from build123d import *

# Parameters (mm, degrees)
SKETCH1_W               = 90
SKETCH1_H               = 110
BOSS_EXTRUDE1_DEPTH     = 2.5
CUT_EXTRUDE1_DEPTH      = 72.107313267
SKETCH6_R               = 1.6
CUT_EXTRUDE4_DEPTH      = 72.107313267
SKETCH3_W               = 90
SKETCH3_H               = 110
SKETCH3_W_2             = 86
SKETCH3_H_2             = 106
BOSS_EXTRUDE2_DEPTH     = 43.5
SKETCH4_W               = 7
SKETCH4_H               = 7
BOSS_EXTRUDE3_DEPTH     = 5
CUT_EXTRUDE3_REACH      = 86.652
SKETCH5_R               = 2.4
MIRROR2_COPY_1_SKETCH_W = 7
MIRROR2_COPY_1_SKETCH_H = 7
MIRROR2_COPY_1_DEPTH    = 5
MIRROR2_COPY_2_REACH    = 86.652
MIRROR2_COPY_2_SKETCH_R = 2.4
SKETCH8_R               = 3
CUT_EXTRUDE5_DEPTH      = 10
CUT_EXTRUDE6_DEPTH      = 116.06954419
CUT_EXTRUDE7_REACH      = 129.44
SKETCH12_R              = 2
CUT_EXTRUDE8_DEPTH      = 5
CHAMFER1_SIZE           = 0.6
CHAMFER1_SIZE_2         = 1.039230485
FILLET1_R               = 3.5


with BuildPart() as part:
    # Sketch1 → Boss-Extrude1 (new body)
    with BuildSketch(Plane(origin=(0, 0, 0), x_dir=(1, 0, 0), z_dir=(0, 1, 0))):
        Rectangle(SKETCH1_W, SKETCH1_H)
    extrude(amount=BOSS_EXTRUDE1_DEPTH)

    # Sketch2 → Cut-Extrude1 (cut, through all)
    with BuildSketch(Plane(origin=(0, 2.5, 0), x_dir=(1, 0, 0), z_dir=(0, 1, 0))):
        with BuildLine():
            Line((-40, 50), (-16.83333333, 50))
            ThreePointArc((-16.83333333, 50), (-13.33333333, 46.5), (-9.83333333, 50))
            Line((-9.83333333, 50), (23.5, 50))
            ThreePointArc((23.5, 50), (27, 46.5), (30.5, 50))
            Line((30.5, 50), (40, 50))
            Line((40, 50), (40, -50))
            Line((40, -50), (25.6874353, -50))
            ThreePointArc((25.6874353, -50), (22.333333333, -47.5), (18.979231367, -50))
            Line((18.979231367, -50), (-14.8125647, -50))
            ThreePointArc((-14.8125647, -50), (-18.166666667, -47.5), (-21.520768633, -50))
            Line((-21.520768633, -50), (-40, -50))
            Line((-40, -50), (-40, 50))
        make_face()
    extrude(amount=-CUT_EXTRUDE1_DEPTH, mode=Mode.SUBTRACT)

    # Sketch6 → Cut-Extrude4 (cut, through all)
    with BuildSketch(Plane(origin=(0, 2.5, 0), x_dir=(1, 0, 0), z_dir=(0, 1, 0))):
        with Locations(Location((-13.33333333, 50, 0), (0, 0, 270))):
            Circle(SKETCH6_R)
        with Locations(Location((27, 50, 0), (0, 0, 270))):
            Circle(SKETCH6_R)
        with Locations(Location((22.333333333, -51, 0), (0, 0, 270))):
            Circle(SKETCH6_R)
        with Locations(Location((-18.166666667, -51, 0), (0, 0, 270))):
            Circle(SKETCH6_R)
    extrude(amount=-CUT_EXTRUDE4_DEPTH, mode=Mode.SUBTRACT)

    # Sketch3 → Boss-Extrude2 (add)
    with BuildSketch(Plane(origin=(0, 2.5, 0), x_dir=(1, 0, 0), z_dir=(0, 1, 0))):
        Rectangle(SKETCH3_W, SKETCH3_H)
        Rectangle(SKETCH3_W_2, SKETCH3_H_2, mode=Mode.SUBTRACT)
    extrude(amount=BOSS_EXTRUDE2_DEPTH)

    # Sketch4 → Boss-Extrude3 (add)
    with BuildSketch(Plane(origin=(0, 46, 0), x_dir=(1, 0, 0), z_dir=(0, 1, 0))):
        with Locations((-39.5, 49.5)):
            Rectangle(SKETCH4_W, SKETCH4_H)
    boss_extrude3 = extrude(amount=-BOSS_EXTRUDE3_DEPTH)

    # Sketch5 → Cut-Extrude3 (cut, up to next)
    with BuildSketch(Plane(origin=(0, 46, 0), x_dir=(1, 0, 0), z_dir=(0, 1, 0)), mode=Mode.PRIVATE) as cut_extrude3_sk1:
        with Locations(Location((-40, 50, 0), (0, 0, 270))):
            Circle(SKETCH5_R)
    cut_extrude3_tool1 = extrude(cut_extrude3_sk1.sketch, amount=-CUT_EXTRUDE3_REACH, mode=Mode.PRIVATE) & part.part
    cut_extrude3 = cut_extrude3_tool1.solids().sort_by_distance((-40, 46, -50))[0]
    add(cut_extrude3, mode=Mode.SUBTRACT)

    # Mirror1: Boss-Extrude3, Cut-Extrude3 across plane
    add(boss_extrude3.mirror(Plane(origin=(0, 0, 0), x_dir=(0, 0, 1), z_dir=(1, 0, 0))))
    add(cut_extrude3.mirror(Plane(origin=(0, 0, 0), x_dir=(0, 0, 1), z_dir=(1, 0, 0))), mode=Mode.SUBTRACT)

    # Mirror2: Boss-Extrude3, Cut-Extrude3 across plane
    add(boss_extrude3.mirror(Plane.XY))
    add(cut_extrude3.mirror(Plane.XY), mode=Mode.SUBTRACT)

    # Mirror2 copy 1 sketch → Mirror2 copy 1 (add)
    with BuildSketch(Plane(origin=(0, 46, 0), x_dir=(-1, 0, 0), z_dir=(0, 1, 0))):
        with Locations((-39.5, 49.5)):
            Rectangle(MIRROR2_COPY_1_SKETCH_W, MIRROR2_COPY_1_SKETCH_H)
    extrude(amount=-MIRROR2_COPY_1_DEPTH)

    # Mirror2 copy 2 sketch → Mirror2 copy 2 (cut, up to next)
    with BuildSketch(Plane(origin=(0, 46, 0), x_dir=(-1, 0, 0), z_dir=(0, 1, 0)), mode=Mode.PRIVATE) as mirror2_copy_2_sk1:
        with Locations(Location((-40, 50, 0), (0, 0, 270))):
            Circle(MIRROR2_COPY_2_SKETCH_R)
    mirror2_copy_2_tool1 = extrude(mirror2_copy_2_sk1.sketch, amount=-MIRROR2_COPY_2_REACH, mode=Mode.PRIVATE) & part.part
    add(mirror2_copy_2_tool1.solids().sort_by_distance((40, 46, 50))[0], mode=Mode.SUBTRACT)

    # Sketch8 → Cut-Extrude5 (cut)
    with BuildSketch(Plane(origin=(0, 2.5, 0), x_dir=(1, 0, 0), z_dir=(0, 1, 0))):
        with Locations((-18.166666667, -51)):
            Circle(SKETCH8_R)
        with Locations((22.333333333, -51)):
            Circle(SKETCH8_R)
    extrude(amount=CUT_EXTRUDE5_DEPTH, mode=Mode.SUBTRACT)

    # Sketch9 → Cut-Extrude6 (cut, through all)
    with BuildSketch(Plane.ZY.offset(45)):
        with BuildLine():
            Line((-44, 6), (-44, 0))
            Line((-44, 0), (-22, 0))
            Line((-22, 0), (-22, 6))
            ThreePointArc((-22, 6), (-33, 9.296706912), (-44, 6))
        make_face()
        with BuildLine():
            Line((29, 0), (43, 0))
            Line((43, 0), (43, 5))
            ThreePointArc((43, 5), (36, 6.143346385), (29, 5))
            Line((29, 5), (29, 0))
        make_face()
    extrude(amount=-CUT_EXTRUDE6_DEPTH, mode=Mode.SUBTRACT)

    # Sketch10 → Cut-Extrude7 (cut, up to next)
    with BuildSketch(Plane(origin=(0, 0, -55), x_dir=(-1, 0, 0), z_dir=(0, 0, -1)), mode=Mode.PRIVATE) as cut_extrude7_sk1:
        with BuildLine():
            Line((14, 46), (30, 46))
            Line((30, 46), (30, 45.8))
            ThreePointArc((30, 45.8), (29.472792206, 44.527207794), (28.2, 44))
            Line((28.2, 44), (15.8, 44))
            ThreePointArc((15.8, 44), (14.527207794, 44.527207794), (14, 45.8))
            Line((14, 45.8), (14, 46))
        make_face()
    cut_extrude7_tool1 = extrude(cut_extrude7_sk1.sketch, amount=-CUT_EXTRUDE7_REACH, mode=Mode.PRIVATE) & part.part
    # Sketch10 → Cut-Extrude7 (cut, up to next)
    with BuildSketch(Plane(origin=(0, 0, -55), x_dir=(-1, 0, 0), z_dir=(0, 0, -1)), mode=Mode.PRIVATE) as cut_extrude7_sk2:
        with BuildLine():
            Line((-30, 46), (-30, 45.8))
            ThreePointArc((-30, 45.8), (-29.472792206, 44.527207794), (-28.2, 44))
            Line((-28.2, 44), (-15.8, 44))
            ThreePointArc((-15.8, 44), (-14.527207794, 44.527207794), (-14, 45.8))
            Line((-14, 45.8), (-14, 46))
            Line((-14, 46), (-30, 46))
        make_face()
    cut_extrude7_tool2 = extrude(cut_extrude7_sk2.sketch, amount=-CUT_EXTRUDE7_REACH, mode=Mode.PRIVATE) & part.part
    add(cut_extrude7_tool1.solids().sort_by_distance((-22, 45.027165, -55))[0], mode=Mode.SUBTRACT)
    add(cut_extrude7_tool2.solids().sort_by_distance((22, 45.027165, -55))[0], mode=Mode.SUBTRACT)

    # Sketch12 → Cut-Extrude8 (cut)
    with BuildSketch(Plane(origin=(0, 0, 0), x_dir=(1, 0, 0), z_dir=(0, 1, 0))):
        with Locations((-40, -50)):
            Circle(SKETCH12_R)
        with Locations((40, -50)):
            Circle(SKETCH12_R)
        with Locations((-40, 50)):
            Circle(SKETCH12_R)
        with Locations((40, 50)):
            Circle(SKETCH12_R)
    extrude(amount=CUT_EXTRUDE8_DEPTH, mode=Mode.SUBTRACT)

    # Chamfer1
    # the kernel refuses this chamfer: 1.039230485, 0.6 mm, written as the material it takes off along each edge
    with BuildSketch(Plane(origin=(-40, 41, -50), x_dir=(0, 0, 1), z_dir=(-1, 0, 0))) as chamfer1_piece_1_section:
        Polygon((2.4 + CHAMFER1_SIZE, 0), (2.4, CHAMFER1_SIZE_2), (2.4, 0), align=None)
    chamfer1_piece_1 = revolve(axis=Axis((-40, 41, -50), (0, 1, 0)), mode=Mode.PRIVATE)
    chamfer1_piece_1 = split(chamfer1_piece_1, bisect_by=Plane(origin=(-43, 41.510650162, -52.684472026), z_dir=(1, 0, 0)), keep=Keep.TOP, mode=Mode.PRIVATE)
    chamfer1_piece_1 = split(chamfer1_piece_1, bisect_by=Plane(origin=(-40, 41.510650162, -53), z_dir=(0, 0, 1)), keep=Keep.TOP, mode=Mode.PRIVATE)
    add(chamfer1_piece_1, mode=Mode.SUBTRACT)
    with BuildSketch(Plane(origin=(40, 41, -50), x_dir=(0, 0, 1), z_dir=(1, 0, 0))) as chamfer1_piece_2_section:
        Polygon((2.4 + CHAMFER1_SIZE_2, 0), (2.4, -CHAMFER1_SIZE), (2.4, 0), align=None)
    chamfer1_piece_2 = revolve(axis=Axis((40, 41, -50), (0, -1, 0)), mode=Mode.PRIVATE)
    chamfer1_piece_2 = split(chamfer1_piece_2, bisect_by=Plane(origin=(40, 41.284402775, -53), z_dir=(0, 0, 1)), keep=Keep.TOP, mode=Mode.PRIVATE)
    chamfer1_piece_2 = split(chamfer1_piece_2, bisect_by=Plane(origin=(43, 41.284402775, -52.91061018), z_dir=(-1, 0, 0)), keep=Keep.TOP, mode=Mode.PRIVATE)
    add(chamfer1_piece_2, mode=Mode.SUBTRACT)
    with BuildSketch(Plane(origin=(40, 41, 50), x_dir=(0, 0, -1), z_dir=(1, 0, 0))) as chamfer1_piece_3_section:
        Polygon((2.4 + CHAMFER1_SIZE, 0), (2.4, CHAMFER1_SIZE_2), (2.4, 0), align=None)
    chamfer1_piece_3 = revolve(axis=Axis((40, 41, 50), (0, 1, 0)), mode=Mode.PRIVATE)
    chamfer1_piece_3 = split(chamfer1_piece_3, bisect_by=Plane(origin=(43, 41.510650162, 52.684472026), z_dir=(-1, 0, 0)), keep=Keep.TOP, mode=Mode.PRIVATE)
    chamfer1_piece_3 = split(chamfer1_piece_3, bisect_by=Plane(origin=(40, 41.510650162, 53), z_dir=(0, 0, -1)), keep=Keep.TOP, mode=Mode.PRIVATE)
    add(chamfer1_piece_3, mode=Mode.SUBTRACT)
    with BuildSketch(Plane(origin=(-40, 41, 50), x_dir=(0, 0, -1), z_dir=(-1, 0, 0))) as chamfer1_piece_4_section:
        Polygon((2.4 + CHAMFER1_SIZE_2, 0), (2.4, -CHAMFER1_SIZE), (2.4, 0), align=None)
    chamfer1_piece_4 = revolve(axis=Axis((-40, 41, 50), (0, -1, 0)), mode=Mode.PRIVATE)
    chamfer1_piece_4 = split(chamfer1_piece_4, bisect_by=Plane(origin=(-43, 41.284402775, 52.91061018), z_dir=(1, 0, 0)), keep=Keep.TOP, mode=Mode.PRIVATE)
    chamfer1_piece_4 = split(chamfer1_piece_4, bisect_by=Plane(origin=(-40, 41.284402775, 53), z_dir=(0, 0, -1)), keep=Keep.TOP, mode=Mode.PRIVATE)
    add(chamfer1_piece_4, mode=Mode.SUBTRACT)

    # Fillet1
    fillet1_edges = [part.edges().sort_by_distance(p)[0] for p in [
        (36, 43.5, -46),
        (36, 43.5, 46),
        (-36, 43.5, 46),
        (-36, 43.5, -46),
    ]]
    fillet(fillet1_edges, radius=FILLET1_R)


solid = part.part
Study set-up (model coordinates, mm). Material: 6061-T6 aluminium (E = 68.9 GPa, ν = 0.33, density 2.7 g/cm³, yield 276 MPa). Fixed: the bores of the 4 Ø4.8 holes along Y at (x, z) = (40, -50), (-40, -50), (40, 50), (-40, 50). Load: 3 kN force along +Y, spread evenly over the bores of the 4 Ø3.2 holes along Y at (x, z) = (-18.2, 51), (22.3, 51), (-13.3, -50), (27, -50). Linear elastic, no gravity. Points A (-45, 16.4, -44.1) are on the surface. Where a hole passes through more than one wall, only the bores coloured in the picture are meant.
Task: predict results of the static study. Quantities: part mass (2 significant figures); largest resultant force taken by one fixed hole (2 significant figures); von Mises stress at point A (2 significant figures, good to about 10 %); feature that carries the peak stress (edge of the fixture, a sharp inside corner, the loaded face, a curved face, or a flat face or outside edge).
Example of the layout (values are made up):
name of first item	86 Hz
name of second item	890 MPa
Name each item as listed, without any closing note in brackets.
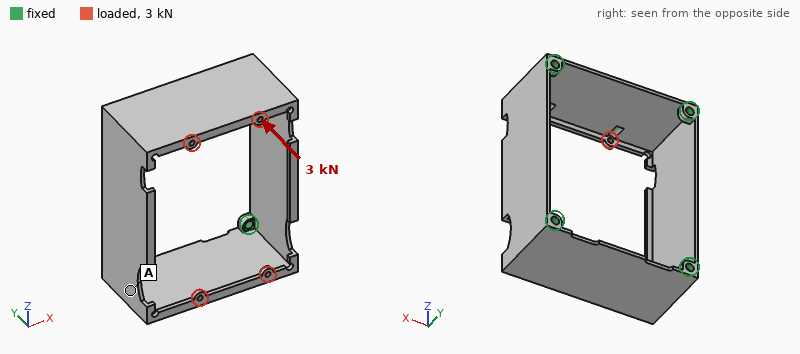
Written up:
part mass	100 g
largest resultant force taken by one fixed hole	940 N
von Mises stress at point A	18 MPa
feature that carries the peak stress	the loaded face
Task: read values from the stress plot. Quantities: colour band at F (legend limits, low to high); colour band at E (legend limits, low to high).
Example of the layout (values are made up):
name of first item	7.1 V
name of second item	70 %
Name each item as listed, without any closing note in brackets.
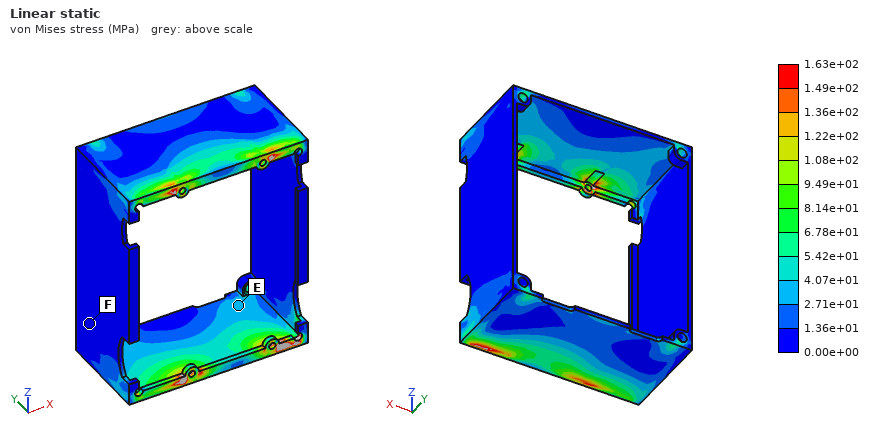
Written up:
colour band at F	0.00e+00 to 1.36e+01 MPa
colour band at E	2.71e+01 to 4.07e+01 MPa
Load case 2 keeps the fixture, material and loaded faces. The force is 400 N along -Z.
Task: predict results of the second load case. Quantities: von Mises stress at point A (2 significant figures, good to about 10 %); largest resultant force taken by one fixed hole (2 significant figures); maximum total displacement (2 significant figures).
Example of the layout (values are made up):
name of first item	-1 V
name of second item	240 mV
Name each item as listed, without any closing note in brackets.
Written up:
von Mises stress at point A	22 MPa
largest resultant force taken by one fixed hole	160 N
maximum total displacement	0.33 mm
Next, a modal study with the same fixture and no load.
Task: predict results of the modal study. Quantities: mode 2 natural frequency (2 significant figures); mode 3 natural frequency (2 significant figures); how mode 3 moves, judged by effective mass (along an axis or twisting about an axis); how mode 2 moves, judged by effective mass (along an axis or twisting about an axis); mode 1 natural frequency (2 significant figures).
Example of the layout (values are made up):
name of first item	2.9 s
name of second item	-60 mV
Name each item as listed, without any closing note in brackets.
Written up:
mode 2 natural frequency	930 Hz
mode 3 natural frequency	1400 Hz
how mode 3 moves, judged by effective mass	along Z
how mode 2 moves, judged by effective mass	along X
mode 1 natural frequency	860 Hz
